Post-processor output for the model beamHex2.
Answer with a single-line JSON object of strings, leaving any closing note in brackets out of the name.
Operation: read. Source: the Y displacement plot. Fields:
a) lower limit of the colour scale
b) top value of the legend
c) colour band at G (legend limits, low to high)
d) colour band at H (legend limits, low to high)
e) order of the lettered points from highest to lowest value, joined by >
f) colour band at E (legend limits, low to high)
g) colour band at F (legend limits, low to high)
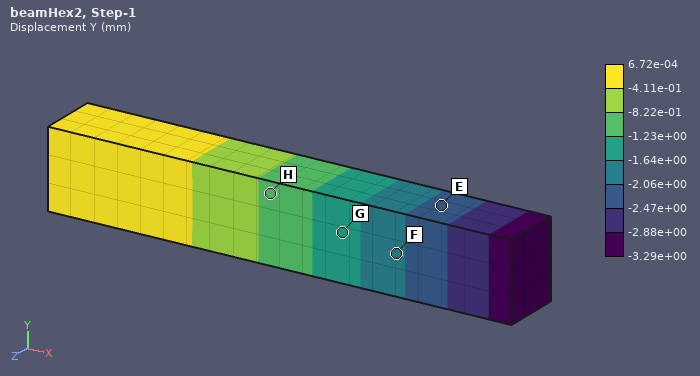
{"lower limit of the colour scale": "-3.29e+00 mm", "top value of the legend": "6.72e-04 mm", "colour band at G": "-1.64e+00 to -1.23e+00 mm", "colour band at H": "-1.23e+00 to -8.22e-01 mm", "order of the lettered points from highest to lowest value, joined by >": "H > G > F > E", "colour band at E": "-2.47e+00 to -2.06e+00 mm", "colour band at F": "-2.06e+00 to -1.64e+00 mm"}
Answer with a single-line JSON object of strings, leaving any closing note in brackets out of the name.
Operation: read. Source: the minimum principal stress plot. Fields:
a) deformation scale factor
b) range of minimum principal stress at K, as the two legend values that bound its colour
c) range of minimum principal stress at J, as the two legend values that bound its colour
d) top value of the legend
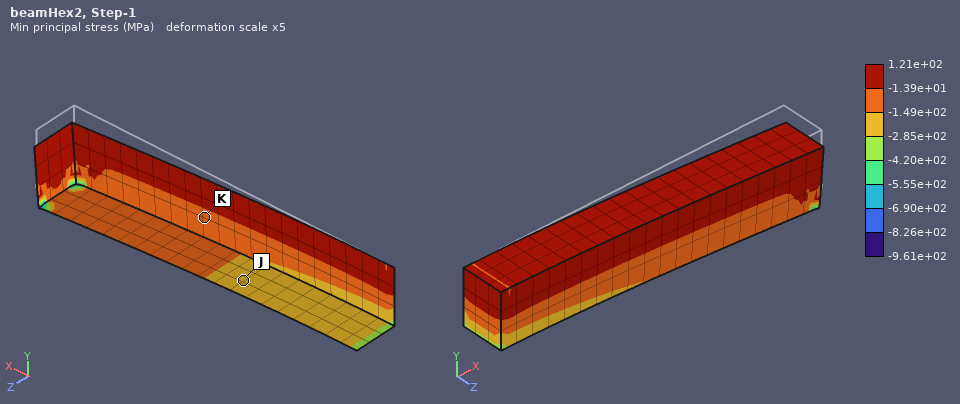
{"deformation scale factor": "5", "range of minimum principal stress at K, as the two legend values that bound its colour": "-1.49e+02 to -1.39e+01 MPa", "range of minimum principal stress at J, as the two legend values that bound its colour": "-2.85e+02 to -1.49e+02 MPa", "top value of the legend": "1.21e+02 MPa"}
